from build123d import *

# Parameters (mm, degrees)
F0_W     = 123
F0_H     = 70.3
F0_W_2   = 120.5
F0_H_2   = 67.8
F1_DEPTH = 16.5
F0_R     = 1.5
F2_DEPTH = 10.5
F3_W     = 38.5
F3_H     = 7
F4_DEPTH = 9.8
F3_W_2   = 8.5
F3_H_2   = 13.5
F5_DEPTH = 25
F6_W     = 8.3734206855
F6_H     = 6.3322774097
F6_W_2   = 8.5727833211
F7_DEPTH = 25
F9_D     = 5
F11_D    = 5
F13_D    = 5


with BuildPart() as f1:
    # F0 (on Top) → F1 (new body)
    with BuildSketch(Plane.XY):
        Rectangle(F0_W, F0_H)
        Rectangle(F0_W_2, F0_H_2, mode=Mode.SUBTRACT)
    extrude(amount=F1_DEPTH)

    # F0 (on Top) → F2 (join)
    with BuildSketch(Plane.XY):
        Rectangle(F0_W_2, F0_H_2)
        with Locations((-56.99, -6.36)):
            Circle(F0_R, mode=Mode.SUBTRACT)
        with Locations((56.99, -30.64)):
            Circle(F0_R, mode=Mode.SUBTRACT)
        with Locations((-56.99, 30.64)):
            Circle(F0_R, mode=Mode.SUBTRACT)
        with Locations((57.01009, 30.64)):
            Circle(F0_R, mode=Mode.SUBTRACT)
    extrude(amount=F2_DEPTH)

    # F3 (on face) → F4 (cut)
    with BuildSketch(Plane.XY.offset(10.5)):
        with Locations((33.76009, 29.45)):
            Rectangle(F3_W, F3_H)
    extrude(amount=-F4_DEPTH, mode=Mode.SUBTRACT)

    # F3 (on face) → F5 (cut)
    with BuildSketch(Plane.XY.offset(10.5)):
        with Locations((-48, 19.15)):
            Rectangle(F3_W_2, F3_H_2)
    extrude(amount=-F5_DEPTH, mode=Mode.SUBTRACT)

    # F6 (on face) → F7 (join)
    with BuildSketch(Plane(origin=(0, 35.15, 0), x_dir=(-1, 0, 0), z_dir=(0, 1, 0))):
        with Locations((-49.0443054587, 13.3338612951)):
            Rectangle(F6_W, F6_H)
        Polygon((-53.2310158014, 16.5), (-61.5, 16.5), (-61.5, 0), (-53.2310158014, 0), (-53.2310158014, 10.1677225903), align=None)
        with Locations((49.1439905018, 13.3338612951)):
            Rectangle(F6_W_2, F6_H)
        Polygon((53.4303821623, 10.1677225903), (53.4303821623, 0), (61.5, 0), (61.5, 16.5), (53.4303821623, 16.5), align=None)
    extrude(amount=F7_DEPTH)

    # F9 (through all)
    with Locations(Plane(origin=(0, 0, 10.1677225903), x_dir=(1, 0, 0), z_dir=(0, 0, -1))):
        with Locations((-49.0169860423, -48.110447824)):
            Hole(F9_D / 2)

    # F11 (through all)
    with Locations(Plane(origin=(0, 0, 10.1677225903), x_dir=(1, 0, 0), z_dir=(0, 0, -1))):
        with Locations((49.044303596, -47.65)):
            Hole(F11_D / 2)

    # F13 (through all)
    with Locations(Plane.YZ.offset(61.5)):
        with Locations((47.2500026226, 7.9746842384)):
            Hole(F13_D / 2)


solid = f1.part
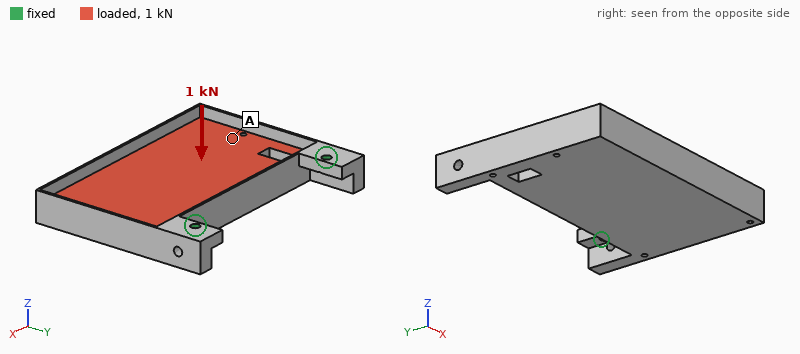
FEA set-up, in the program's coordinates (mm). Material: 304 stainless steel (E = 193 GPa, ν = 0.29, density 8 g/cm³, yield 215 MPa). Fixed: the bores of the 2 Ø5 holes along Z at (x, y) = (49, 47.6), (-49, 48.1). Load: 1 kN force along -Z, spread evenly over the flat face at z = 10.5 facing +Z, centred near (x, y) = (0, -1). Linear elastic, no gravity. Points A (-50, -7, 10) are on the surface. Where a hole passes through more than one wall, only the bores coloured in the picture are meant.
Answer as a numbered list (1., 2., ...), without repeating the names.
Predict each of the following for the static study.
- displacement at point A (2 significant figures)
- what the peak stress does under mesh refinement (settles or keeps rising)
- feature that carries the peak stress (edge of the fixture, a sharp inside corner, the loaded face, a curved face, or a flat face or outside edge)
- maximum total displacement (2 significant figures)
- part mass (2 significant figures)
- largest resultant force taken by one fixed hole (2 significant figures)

1. 0.13 mm
2. keeps rising
3. edge of the fixture
4. 0.21 mm
5. 790 g
6. 530 N
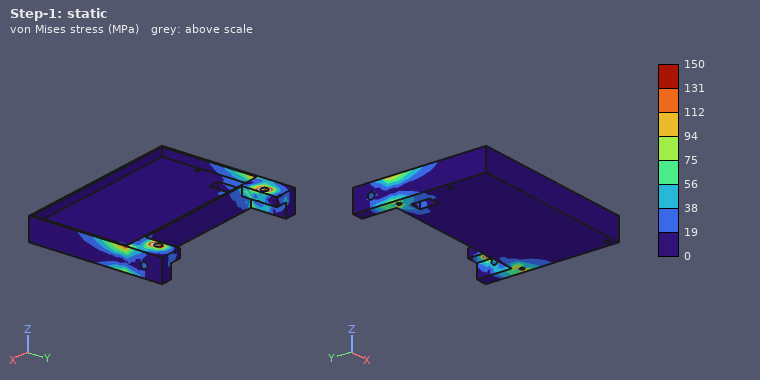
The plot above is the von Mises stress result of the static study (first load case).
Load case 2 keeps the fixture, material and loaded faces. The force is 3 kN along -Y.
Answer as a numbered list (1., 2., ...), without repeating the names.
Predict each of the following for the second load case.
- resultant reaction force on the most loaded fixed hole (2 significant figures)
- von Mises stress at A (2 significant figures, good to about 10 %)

1. 1.6 kN
2. 6.8 MPa
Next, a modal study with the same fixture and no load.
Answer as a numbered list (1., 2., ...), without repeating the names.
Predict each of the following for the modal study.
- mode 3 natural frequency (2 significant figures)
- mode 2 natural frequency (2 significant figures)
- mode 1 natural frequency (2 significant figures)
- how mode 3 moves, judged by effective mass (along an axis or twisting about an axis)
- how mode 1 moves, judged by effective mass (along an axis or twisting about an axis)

1. 2200 Hz
2. 1600 Hz
3. 500 Hz
4. along X
5. along Z
